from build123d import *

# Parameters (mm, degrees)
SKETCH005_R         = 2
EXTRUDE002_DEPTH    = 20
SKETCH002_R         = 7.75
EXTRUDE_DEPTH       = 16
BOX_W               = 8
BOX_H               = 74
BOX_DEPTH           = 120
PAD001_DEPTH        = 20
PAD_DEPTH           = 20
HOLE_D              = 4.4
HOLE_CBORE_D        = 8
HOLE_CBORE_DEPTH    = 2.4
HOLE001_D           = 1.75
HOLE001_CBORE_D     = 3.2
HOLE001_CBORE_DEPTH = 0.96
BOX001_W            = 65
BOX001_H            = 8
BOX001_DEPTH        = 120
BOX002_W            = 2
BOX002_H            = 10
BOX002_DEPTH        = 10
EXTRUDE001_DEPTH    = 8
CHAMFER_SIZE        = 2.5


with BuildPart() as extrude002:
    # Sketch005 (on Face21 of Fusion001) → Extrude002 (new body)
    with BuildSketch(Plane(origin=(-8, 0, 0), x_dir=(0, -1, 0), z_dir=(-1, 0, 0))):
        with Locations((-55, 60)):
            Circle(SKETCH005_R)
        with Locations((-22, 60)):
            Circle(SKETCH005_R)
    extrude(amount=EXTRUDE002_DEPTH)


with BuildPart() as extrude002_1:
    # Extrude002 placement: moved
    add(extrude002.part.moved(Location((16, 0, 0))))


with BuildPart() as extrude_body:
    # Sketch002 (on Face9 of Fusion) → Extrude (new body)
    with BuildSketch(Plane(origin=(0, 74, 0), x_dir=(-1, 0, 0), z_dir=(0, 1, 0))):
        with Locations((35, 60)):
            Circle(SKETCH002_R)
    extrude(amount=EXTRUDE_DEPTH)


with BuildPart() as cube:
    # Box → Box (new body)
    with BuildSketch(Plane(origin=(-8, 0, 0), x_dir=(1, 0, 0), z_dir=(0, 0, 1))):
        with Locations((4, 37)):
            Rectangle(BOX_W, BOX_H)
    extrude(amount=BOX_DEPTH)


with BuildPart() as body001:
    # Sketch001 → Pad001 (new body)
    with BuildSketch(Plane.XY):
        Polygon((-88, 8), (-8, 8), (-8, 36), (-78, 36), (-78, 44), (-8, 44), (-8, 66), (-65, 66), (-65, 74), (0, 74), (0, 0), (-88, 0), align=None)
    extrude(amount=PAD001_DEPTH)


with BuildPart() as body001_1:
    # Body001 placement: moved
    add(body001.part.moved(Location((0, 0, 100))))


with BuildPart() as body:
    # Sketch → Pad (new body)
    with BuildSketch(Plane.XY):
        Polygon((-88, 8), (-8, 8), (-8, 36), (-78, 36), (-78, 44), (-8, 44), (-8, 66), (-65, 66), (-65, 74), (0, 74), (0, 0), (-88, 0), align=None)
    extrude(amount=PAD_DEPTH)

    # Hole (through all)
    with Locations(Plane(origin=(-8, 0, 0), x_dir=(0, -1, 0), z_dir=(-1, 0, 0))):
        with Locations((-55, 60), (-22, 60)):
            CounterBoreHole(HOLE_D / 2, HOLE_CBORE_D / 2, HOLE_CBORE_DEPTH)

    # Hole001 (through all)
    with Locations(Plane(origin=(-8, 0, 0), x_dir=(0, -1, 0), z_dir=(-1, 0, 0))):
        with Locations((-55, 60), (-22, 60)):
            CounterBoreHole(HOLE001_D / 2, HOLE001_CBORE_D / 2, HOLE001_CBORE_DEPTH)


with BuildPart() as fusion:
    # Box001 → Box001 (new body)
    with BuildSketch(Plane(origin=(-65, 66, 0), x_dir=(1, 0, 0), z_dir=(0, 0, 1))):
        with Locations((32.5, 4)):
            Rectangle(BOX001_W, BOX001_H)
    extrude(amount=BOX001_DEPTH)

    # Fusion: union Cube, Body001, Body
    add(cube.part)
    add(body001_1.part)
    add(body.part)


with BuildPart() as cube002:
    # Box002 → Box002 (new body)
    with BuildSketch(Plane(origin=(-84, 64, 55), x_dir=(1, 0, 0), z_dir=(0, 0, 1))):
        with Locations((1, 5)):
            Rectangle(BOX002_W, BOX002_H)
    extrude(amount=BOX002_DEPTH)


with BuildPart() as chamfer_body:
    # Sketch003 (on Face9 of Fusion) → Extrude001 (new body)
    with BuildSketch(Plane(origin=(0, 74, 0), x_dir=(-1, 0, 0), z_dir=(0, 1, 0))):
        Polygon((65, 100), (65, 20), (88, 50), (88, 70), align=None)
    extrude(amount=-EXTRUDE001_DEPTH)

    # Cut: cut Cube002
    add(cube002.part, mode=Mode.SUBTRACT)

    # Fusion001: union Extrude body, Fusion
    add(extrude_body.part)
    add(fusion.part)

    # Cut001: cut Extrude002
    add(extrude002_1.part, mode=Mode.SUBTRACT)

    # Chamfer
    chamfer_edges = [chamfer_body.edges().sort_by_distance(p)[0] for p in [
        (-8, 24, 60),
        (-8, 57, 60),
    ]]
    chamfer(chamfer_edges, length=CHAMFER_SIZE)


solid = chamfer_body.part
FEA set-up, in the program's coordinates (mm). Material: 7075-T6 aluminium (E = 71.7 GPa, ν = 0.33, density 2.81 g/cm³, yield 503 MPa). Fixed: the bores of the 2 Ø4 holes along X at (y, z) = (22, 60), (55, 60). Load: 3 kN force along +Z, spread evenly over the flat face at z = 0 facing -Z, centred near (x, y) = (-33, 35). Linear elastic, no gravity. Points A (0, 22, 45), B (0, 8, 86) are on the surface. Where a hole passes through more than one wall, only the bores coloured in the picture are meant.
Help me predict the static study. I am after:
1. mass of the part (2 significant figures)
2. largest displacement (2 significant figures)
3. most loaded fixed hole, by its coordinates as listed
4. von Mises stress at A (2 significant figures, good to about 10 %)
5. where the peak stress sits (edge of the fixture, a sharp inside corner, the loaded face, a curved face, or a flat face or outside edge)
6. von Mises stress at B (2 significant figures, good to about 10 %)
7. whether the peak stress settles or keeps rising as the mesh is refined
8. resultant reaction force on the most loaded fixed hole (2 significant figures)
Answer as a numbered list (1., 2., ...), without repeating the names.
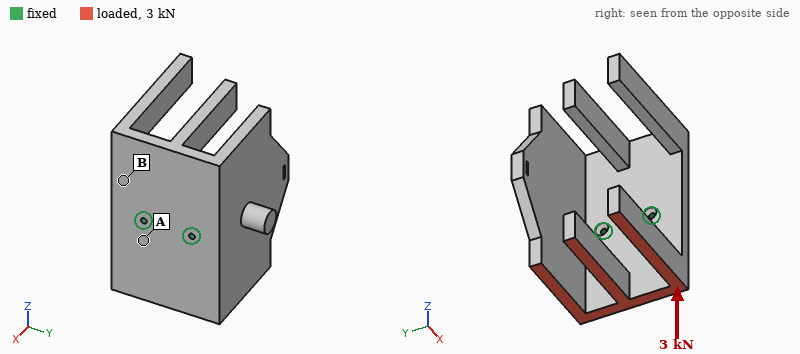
1. 520 g
2. 1.9 mm
3. (22, 60)
4. 56 MPa
5. edge of the fixture
6. 21 MPa
7. keeps rising
8. 1.8 kN
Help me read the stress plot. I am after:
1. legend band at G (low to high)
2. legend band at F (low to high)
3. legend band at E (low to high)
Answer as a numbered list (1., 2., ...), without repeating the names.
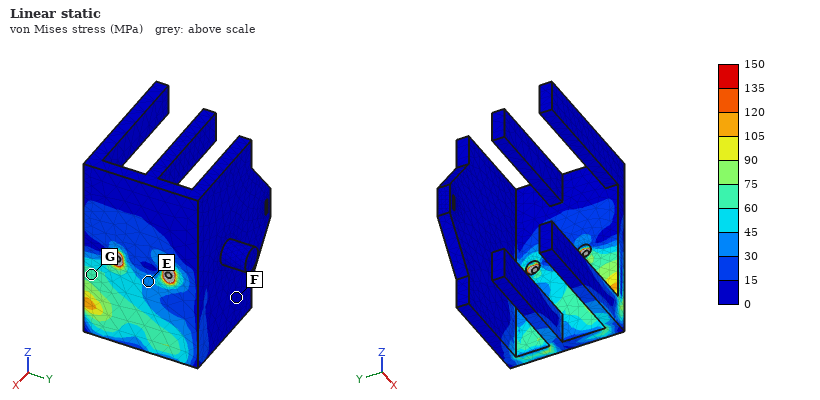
1. 60 to 75 MPa
2. 0 to 15 MPa
3. 30 to 45 MPa
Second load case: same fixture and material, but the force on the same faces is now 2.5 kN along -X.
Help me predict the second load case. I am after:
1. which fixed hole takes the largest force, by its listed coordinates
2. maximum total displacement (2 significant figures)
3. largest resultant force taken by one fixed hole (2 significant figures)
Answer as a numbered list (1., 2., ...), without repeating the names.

1. (22, 60)
2. 2.0 mm
3. 1.5 kN
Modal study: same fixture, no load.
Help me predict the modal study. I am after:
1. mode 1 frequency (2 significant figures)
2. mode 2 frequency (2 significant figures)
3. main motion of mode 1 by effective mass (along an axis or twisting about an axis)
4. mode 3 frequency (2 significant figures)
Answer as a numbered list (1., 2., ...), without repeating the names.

1. 460 Hz
2. 650 Hz
3. along Z
4. 650 Hz
